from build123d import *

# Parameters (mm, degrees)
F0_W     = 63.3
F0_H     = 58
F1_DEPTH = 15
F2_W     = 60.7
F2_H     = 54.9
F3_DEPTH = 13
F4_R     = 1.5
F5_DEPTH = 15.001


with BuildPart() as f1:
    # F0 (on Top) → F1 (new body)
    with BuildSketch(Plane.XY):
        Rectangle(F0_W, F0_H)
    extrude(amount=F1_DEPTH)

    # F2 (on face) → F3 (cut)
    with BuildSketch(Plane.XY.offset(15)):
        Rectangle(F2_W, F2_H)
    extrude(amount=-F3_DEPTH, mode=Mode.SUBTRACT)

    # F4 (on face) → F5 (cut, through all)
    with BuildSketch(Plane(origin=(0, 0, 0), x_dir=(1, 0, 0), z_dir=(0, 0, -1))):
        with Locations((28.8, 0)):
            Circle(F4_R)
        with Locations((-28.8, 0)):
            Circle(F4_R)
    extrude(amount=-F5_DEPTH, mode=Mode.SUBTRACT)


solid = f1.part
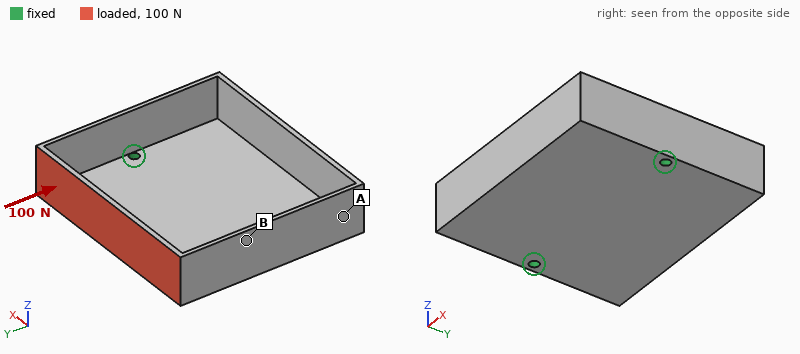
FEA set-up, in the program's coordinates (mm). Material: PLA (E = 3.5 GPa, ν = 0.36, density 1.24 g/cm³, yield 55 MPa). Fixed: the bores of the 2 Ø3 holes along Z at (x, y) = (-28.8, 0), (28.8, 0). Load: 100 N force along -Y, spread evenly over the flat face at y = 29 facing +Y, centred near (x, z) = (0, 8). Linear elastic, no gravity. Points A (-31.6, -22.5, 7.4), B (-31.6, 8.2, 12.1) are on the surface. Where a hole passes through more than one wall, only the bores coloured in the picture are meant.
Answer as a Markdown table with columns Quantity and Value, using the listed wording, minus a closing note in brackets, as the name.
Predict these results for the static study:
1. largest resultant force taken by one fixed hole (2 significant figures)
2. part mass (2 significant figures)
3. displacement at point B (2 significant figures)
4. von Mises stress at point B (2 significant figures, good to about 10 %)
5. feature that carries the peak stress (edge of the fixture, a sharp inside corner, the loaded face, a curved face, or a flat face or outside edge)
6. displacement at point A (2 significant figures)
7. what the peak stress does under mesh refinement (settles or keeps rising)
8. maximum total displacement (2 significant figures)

| Quantity | Value |
|---|---|
| largest resultant force taken by one fixed hole | 51 N |
| part mass | 15 g |
| displacement at point B | 0.16 mm |
| von Mises stress at point B | 4.1 MPa |
| feature that carries the peak stress | edge of the fixture |
| displacement at point A | 0.25 mm |
| what the peak stress does under mesh refinement | keeps rising |
| maximum total displacement | 0.92 mm |
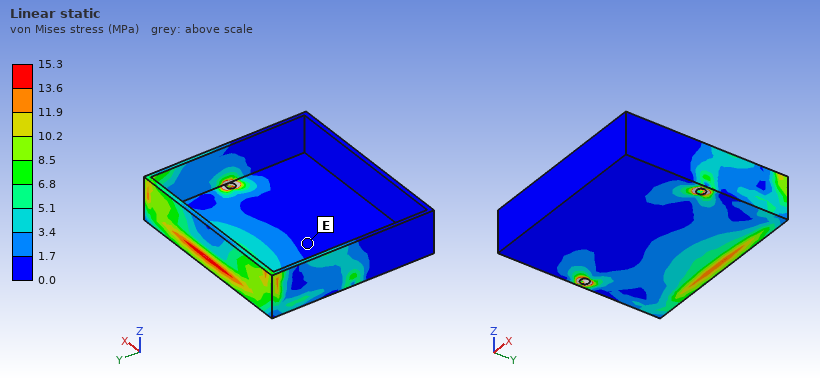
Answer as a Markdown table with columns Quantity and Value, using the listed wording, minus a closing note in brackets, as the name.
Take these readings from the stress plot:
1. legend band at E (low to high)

| Quantity | Value |
|---|---|
| legend band at E | 0.0 to 1.7 MPa |
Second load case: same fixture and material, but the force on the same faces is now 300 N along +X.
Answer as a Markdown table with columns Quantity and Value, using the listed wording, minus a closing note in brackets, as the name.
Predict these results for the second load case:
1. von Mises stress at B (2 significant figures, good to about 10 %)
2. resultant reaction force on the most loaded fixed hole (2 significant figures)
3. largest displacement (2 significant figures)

| Quantity | Value |
|---|---|
| von Mises stress at B | 8.2 MPa |
| resultant reaction force on the most loaded fixed hole | 220 N |
| largest displacement | 1.0 mm |
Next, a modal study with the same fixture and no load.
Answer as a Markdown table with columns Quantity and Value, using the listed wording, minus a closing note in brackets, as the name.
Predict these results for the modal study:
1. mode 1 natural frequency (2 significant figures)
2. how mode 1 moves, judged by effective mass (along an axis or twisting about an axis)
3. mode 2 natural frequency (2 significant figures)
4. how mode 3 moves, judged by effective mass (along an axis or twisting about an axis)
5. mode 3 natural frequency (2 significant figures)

| Quantity | Value |
|---|---|
| mode 1 natural frequency | 500 Hz |
| how mode 1 moves, judged by effective mass | twisting about X |
| mode 2 natural frequency | 800 Hz |
| how mode 3 moves, judged by effective mass | along Z |
| mode 3 natural frequency | 1200 Hz |
